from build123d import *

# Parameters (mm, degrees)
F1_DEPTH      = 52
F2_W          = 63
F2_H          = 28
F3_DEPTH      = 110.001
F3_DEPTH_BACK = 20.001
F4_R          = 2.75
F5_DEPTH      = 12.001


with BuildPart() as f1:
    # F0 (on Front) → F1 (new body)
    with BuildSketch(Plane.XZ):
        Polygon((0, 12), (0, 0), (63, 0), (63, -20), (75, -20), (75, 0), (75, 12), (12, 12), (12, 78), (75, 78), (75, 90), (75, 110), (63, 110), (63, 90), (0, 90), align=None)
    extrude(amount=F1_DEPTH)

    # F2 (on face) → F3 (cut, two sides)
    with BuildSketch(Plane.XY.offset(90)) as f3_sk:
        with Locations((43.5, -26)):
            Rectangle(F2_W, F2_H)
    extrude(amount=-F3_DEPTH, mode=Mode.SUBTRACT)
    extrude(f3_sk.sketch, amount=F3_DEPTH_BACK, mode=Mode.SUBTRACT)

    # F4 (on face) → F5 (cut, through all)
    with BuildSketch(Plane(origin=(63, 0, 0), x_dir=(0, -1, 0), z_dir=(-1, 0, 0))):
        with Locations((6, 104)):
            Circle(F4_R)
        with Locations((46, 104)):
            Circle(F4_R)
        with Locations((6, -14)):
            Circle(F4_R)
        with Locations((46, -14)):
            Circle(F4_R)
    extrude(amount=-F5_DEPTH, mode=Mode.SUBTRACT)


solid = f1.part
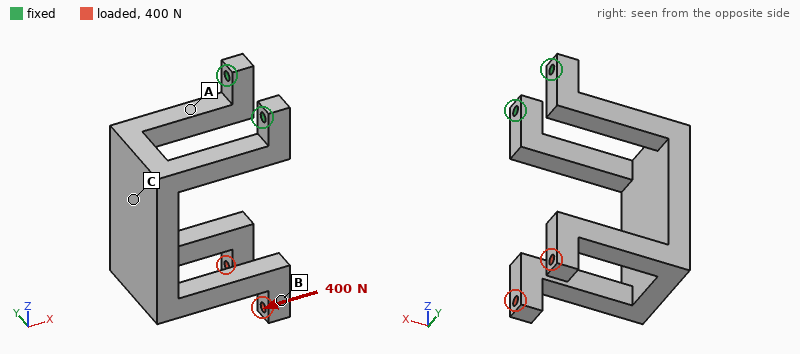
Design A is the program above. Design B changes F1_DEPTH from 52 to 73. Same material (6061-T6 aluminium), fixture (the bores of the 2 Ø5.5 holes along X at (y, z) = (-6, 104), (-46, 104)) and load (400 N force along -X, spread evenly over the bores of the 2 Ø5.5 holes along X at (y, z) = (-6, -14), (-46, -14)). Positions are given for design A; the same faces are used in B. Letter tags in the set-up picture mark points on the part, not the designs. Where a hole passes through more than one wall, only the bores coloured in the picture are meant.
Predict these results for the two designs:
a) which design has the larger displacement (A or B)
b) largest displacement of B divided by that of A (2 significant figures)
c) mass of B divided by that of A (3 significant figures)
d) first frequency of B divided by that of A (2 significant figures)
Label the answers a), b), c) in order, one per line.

a) A
b) 0.63
c) 1.63
d) 1.0
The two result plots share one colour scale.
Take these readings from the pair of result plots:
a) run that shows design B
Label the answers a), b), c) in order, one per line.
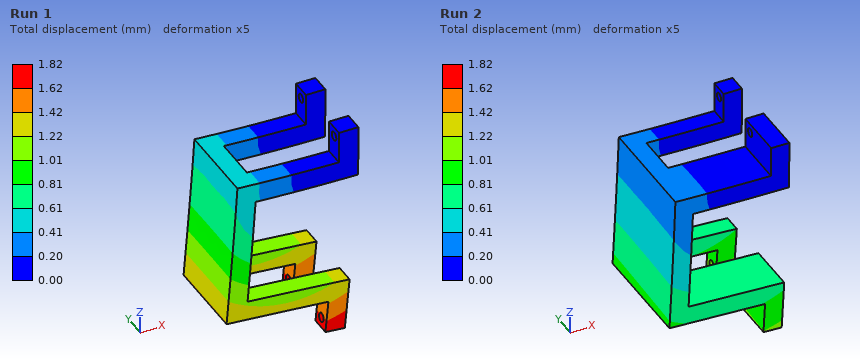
a) Run 2
